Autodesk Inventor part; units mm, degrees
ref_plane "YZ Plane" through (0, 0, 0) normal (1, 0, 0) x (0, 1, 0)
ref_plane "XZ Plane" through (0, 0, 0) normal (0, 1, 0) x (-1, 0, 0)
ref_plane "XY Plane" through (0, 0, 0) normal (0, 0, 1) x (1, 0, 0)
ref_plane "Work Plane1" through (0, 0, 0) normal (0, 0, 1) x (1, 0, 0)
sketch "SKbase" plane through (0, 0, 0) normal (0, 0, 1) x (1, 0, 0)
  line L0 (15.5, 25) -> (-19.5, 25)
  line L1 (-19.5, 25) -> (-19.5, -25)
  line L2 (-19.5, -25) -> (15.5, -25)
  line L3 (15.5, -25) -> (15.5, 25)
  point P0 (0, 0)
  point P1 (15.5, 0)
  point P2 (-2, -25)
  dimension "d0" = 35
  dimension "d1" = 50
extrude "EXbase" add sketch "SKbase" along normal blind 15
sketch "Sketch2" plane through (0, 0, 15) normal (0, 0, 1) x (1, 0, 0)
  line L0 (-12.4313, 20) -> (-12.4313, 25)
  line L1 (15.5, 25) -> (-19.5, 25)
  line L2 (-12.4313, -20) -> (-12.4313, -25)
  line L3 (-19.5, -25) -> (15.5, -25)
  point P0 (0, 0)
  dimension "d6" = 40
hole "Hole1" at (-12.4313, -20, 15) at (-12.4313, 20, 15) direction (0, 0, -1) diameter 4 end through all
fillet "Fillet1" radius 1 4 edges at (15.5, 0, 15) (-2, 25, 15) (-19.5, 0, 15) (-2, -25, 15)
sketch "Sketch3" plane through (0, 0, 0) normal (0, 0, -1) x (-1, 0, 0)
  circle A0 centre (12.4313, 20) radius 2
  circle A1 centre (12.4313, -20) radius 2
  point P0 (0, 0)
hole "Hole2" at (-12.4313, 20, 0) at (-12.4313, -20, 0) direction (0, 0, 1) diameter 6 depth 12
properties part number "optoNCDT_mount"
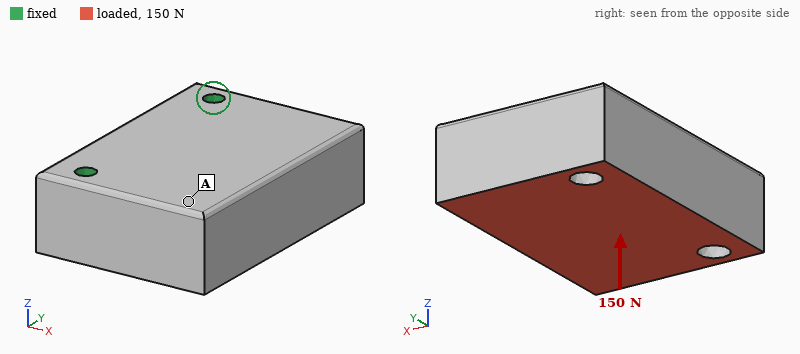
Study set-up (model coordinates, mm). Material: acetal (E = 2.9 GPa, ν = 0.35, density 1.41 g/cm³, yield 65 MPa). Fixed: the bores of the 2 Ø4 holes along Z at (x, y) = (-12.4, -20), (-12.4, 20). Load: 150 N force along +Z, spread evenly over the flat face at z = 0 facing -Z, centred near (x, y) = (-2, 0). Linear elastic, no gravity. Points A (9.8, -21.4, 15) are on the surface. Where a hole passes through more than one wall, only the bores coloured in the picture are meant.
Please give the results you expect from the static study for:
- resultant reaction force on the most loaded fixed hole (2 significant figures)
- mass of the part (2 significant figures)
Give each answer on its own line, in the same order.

78 N
36 g
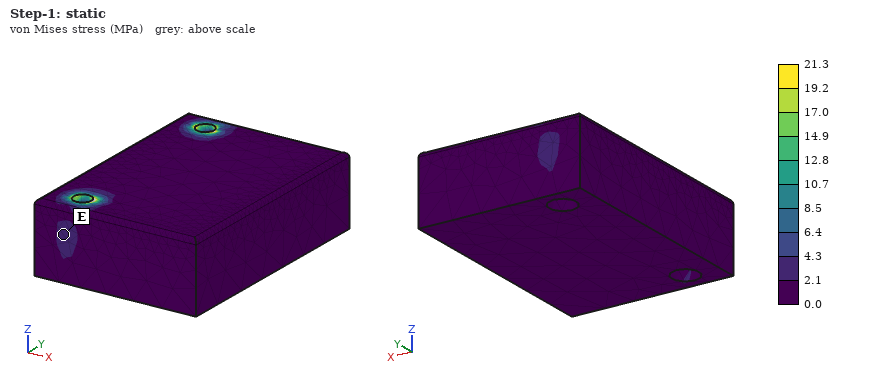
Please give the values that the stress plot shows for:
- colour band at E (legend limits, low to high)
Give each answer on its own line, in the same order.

2.1 to 4.3 MPa
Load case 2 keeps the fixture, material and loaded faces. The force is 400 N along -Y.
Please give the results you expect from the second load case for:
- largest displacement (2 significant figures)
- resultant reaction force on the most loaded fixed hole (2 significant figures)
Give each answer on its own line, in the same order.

38 µm
260 N
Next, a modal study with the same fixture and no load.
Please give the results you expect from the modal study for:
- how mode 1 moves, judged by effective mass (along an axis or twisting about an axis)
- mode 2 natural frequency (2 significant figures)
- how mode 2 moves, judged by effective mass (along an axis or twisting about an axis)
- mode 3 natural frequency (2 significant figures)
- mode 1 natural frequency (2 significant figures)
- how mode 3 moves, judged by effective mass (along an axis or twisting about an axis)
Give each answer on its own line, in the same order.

along Z
3300 Hz
along Y
3900 Hz
750 Hz
along Y
